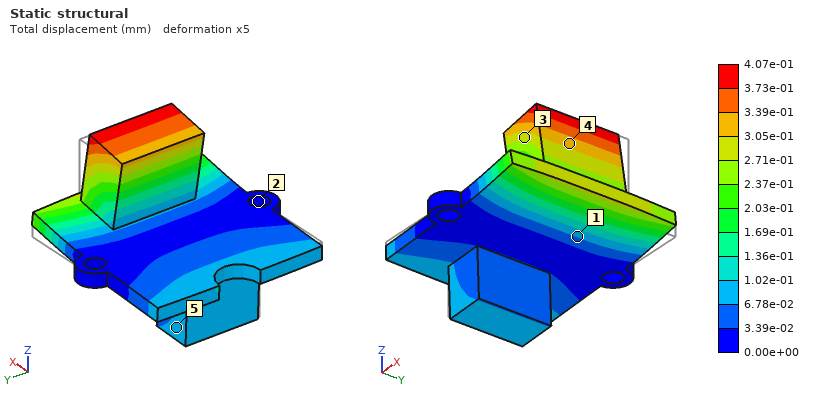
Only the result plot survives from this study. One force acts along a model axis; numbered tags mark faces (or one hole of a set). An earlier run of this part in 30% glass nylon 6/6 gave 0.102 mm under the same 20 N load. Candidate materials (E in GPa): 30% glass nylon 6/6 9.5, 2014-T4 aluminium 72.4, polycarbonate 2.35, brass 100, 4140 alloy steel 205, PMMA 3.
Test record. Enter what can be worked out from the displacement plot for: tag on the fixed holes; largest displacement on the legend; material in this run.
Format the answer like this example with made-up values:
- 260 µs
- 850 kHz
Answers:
- 2
- 4.07e-01 mm
- polycarbonate
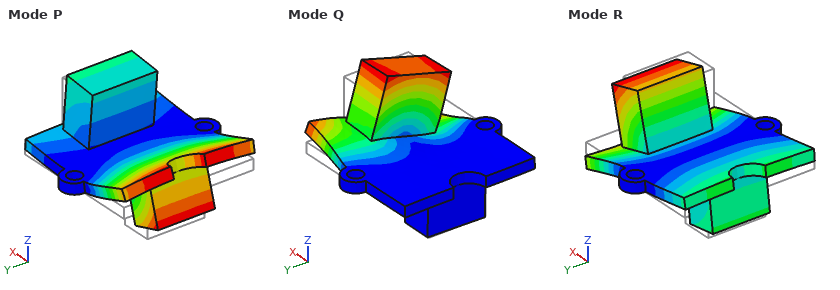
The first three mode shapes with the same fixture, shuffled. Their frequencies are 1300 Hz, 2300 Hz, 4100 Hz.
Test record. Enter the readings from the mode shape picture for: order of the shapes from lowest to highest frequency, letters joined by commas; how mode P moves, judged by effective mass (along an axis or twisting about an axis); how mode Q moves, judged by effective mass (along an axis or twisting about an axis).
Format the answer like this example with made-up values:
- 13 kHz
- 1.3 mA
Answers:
- R, P, Q
- along Z
- along Y
